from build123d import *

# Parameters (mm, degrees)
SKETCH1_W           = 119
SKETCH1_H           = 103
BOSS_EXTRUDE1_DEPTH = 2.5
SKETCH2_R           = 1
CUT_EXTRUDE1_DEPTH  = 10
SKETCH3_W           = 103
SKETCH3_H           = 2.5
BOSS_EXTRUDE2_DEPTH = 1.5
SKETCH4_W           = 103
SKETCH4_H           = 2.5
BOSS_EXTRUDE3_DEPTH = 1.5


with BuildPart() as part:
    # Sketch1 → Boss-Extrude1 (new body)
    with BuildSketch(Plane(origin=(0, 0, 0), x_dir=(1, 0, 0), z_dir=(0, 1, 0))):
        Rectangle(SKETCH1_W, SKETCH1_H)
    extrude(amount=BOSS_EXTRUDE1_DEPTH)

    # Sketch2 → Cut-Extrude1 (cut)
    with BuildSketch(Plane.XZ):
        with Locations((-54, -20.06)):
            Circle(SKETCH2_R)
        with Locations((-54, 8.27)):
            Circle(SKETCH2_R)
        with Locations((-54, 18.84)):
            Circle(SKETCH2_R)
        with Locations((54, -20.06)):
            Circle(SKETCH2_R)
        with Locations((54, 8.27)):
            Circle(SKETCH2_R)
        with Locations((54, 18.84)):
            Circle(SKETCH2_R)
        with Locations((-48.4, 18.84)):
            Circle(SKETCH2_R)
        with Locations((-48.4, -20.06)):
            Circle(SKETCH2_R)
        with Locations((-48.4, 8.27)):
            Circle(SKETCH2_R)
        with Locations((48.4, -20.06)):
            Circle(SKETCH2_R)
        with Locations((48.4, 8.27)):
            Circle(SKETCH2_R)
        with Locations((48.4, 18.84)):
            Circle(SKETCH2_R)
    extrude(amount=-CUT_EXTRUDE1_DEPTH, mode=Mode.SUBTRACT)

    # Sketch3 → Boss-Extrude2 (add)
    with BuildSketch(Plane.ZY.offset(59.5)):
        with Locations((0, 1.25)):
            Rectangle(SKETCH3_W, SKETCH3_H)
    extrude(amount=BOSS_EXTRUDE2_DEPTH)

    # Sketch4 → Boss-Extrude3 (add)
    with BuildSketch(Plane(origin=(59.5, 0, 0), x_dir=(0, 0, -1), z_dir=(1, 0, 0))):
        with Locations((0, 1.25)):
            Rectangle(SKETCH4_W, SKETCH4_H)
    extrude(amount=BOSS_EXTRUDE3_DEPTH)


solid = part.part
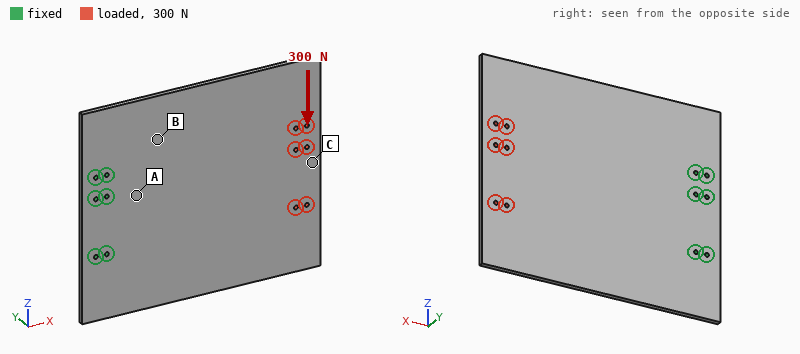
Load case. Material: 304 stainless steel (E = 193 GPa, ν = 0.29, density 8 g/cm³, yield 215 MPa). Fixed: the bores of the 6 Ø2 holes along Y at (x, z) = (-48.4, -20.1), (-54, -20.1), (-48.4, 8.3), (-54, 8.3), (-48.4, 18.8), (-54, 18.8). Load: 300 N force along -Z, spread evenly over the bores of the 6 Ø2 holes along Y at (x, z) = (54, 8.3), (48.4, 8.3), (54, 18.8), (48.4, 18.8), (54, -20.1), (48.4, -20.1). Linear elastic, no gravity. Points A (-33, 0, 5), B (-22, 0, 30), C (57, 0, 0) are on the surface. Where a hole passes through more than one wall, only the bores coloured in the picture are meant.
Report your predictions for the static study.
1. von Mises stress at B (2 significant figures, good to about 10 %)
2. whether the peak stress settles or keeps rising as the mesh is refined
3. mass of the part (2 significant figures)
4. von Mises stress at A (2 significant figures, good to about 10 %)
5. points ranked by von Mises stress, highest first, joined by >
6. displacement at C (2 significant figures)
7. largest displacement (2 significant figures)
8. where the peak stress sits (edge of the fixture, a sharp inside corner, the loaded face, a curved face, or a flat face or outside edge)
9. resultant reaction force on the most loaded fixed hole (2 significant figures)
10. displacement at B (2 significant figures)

4.3 MPa
keeps rising
250 g
8.6 MPa
A > B > C
12 µm
14 µm
edge of the fixture
520 N
4.0 µm
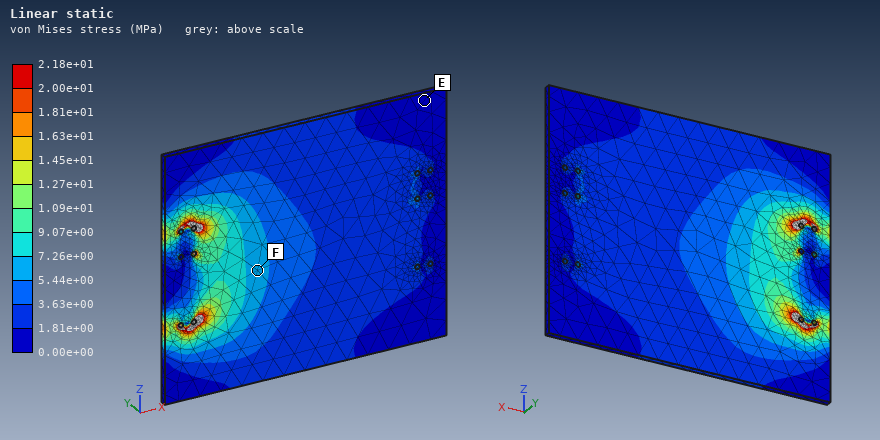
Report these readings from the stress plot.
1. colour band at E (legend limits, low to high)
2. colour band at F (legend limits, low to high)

0.00e+00 to 1.81e+00 MPa
5.44e+00 to 7.26e+00 MPa
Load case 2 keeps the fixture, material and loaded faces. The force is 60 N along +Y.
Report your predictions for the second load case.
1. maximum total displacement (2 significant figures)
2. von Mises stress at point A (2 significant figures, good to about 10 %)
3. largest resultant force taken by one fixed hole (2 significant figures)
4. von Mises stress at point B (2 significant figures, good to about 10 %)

0.97 mm
49 MPa
230 N
39 MPa
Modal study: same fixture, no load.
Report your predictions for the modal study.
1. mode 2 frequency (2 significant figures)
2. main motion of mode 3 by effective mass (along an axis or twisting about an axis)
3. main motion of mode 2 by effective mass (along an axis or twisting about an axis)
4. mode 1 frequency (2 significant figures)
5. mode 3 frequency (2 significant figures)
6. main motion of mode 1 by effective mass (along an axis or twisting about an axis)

380 Hz
along Y
twisting about X
160 Hz
920 Hz
along Y
